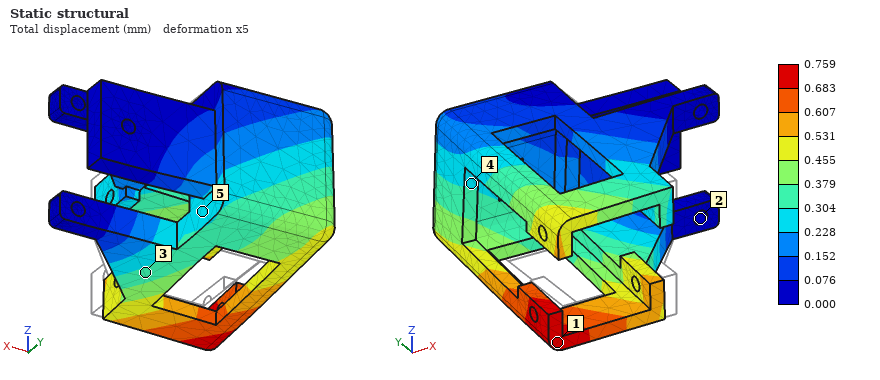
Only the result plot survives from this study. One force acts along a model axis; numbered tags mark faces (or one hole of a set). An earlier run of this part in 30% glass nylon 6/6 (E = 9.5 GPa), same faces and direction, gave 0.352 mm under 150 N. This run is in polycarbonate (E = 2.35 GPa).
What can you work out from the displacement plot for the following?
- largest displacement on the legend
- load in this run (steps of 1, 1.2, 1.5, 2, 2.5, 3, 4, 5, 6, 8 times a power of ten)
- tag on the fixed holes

0.759 mm
80 N
2
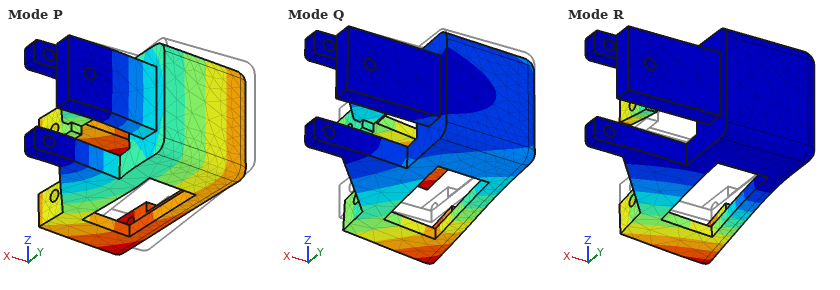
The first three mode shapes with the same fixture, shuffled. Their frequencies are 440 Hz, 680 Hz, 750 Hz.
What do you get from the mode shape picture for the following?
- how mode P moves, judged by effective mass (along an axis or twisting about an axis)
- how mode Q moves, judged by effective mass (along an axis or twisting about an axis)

along Y
along Z
